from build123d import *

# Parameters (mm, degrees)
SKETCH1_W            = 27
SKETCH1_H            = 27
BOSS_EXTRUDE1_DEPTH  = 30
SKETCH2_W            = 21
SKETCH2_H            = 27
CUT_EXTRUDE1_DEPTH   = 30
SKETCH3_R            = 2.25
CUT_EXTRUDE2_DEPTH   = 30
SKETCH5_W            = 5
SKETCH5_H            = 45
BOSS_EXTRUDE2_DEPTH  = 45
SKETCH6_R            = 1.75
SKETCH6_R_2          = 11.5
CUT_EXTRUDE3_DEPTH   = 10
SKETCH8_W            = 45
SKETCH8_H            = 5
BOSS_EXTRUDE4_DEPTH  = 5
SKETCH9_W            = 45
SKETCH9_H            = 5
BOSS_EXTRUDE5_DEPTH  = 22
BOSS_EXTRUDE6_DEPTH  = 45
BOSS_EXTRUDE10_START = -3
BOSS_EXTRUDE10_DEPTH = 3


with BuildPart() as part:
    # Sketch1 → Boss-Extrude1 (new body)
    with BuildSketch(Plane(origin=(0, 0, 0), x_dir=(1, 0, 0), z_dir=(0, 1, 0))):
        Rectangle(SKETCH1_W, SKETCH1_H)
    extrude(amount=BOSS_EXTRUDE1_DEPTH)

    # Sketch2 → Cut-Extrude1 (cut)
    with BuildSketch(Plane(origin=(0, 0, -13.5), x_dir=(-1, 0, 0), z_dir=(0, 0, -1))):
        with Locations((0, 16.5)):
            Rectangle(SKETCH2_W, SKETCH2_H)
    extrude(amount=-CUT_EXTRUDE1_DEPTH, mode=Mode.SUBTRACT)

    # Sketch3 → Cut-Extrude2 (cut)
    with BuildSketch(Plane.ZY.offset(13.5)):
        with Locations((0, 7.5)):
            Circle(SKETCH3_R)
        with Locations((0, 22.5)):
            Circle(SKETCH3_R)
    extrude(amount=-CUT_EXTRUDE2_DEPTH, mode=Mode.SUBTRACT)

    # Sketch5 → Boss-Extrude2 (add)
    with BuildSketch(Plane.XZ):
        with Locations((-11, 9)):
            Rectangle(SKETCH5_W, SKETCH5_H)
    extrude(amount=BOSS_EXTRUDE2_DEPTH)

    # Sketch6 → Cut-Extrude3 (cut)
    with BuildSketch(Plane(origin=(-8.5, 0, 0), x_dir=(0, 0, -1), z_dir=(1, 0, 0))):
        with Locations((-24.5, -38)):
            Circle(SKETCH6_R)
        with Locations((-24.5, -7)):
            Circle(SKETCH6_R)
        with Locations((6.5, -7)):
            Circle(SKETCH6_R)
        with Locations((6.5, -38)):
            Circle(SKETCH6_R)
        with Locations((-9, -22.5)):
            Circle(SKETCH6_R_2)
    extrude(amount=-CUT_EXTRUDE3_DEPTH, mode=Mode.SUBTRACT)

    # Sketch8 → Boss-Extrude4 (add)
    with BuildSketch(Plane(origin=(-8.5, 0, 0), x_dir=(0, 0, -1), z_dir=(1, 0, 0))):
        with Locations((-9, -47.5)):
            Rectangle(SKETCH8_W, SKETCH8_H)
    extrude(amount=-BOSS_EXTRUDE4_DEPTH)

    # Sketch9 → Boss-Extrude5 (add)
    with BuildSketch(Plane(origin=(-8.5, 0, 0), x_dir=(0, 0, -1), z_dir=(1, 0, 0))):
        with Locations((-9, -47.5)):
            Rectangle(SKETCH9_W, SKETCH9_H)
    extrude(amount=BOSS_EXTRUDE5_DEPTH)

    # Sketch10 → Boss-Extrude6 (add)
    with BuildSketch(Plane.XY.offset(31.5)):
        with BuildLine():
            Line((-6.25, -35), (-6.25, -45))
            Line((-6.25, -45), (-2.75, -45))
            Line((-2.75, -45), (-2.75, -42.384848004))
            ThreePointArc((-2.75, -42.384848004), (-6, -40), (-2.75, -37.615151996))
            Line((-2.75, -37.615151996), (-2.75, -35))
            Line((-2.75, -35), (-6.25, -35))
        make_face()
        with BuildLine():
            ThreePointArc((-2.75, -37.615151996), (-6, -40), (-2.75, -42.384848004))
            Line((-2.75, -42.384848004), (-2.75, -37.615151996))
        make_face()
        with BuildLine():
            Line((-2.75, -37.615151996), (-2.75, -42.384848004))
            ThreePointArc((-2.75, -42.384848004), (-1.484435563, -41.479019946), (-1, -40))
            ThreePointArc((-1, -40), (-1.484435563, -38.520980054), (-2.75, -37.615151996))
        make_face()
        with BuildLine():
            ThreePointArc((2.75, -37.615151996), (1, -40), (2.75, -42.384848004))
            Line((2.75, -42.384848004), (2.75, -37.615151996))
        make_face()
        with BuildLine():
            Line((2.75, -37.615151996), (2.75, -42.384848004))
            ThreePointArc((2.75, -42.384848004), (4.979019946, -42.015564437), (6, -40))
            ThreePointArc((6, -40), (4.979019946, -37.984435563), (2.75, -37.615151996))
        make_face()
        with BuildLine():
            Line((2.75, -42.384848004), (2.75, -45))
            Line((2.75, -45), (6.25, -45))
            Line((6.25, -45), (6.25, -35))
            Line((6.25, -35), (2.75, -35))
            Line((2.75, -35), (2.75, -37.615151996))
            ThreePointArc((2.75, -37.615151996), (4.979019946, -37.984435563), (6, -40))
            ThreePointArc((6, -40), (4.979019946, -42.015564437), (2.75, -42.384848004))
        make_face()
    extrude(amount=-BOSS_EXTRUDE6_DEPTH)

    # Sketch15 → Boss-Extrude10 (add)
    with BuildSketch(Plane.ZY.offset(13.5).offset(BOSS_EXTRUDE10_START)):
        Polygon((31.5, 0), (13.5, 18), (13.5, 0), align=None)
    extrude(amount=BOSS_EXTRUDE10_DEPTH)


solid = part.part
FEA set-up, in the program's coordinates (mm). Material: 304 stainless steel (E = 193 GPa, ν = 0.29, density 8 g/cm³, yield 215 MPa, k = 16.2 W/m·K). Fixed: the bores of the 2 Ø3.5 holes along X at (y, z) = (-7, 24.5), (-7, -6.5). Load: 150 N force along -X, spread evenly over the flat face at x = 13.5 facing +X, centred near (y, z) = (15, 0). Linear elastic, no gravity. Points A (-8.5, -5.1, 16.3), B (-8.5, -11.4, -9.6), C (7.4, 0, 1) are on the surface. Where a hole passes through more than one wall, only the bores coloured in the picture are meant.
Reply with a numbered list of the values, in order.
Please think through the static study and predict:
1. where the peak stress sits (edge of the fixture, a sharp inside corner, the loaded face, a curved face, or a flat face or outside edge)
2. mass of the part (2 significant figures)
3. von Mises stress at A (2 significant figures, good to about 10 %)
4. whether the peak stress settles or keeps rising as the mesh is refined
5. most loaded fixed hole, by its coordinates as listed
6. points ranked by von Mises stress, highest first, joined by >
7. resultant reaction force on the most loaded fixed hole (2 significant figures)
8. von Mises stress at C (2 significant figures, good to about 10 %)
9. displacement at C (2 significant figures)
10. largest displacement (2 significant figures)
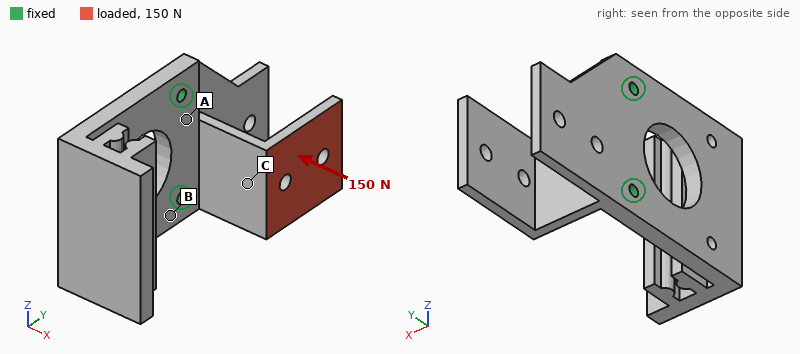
1. edge of the fixture
2. 200 g
3. 11 MPa
4. keeps rising
5. (-7, -6.5)
6. C > A > B
7. 110 N
8. 41 MPa
9. 0.032 mm
10. 0.16 mm
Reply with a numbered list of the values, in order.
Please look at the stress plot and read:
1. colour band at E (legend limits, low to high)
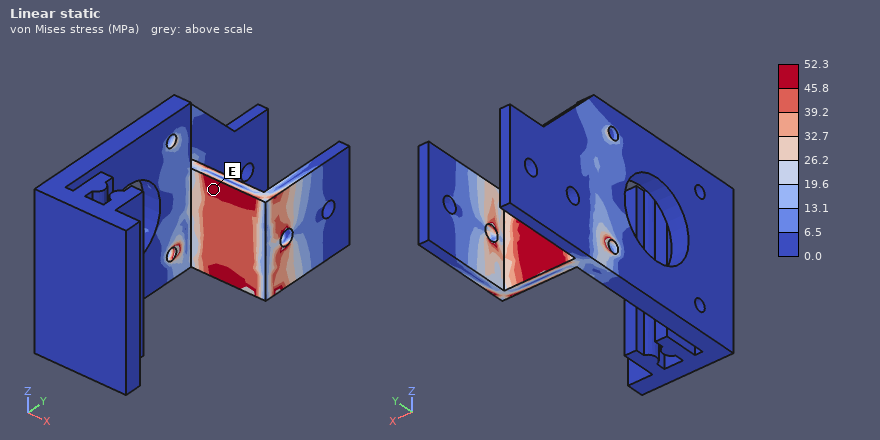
1. 45.8 to 52.3 MPa
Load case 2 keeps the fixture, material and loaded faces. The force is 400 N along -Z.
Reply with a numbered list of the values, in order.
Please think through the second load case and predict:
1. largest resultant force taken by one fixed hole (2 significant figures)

1. 470 N
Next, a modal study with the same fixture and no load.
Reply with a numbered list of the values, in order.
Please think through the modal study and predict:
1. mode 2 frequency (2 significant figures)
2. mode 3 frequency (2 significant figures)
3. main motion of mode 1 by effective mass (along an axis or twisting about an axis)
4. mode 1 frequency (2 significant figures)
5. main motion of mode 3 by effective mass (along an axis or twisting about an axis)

1. 1200 Hz
2. 1800 Hz
3. along X
4. 800 Hz
5. along Z
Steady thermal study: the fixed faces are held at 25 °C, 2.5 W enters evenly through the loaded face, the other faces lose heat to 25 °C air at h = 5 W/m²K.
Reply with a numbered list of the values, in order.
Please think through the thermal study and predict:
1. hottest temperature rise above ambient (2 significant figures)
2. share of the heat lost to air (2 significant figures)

1. 65 K
2. 24 %
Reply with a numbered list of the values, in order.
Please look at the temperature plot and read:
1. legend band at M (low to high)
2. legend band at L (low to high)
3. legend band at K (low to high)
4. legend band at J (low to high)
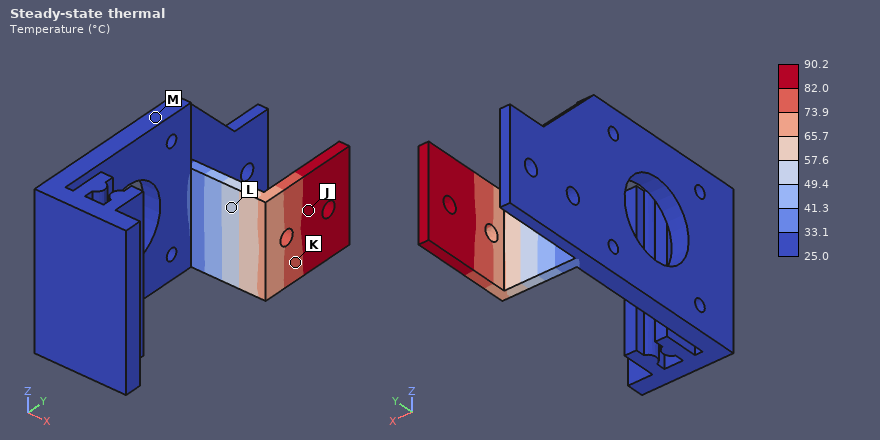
1. 25.0 to 33.1 °C
2. 49.4 to 57.6 °C
3. 73.9 to 82.0 °C
4. 82.0 to 90.2 °C
